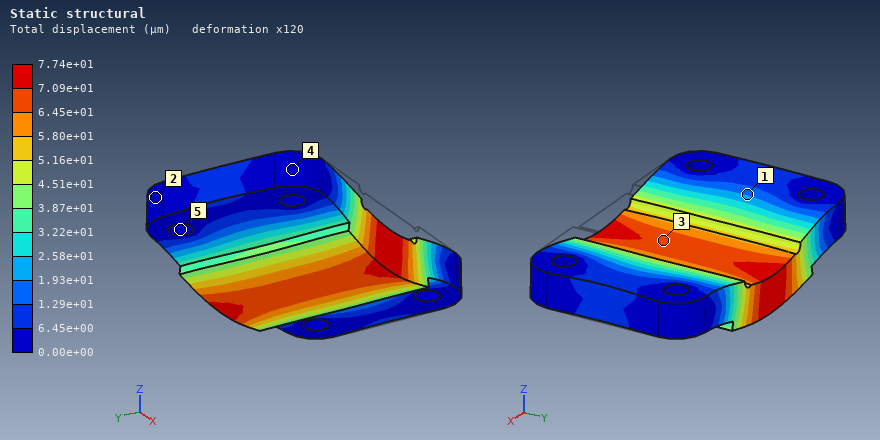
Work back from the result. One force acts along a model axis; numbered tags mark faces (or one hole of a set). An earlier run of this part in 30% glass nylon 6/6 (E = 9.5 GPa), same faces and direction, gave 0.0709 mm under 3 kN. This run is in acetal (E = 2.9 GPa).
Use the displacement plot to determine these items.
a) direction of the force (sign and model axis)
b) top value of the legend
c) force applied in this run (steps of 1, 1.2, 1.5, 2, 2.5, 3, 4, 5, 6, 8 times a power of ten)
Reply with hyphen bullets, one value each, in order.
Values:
- -Z
- 7.74e+01 µm
- 1 kN
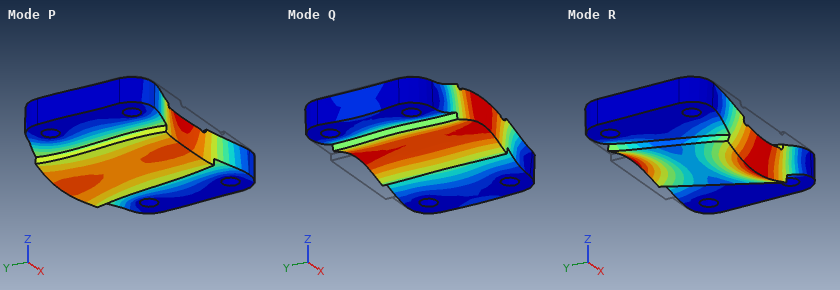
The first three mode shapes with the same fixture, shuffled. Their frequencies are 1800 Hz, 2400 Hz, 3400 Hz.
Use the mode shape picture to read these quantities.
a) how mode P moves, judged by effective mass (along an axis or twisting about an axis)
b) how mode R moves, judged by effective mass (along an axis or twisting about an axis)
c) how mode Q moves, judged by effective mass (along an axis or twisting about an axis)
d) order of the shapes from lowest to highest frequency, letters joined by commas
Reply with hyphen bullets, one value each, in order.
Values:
- along Y
- twisting about X
- along Z
- Q, R, P
